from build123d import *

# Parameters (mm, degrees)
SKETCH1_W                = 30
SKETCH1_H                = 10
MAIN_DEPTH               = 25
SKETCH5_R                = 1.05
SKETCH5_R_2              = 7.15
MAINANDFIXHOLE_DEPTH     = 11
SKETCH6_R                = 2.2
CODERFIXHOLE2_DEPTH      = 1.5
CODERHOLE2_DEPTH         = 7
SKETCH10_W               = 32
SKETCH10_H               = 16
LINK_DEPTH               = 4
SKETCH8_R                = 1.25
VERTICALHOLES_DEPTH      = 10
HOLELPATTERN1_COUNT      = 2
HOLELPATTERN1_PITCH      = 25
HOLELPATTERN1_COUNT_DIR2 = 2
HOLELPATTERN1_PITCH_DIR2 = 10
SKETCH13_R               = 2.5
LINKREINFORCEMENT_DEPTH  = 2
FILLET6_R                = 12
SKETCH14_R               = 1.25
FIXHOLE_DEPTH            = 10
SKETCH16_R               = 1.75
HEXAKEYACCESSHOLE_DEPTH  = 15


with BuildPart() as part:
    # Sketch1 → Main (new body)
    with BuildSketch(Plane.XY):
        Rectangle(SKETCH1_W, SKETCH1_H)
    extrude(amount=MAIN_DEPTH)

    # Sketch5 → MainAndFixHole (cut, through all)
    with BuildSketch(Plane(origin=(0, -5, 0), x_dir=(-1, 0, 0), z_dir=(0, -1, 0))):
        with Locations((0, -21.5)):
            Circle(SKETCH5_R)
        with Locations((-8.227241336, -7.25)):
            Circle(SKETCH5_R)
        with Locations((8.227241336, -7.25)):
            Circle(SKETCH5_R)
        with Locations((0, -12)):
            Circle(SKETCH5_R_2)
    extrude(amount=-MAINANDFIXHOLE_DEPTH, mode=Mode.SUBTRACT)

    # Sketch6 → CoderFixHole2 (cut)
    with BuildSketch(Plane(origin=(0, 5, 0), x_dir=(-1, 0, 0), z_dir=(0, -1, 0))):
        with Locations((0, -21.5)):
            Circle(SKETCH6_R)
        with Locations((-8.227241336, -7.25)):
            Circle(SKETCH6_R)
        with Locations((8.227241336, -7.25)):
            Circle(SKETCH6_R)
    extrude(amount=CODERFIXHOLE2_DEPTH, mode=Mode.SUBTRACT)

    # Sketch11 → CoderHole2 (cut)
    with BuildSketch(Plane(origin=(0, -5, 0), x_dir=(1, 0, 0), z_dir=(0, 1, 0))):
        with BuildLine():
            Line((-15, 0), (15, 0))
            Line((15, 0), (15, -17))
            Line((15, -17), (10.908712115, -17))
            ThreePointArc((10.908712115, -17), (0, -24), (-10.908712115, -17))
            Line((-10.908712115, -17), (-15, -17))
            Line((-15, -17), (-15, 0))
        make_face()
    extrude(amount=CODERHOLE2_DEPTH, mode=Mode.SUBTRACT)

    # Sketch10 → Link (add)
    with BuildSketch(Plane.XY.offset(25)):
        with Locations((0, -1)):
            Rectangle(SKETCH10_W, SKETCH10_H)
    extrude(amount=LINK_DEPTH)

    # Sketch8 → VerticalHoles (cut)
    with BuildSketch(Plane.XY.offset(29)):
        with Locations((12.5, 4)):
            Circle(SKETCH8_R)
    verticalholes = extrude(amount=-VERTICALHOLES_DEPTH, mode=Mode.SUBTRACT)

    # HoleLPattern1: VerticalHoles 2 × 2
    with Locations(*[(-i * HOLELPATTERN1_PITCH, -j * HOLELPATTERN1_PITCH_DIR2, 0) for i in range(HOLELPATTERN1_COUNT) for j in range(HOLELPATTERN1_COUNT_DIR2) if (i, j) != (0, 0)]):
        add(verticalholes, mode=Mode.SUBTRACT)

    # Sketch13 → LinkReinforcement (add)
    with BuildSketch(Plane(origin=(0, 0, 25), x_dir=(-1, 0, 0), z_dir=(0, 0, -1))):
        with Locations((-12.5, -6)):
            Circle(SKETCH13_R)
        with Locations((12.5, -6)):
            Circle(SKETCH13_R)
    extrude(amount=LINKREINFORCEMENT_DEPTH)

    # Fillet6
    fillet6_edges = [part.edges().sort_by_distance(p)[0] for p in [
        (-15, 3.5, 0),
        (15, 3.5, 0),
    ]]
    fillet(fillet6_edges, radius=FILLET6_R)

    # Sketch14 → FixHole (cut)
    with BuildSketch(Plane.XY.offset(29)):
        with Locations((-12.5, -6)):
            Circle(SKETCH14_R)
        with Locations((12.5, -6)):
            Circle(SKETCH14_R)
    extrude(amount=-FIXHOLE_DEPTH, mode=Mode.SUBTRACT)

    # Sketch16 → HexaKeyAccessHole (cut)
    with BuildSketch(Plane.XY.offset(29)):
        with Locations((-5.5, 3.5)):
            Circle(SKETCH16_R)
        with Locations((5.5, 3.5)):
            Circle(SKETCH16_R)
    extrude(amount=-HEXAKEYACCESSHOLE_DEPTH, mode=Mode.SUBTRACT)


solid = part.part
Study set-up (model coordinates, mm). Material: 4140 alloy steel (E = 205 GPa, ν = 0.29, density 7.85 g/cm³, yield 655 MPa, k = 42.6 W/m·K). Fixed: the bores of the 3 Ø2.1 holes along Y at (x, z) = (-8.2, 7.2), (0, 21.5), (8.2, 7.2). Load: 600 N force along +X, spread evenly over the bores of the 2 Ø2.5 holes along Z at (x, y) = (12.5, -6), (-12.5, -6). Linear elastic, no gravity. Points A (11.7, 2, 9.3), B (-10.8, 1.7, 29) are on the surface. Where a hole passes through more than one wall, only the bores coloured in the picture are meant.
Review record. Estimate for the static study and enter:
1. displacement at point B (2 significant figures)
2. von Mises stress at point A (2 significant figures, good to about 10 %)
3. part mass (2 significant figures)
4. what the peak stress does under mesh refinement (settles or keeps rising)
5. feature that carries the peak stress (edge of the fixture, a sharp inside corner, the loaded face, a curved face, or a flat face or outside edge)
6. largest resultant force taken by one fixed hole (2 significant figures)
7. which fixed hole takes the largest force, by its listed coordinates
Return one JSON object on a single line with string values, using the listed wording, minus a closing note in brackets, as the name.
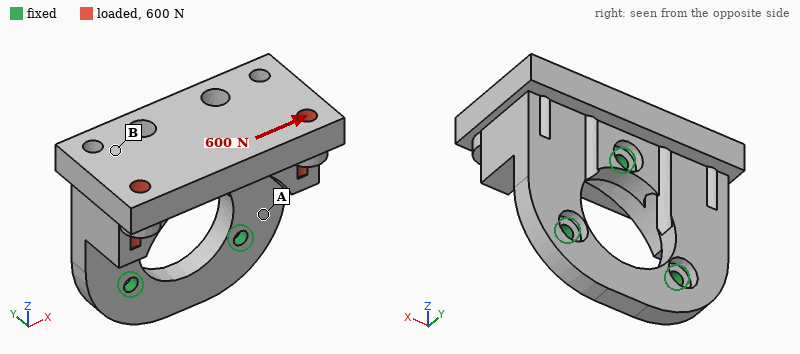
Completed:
{"displacement at point B": "23 µm", "von Mises stress at point A": "50 MPa", "part mass": "32 g", "what the peak stress does under mesh refinement": "keeps rising", "feature that carries the peak stress": "edge of the fixture", "largest resultant force taken by one fixed hole": "490 N", "which fixed hole takes the largest force, by its listed coordinates": "(0, 21.5)"}
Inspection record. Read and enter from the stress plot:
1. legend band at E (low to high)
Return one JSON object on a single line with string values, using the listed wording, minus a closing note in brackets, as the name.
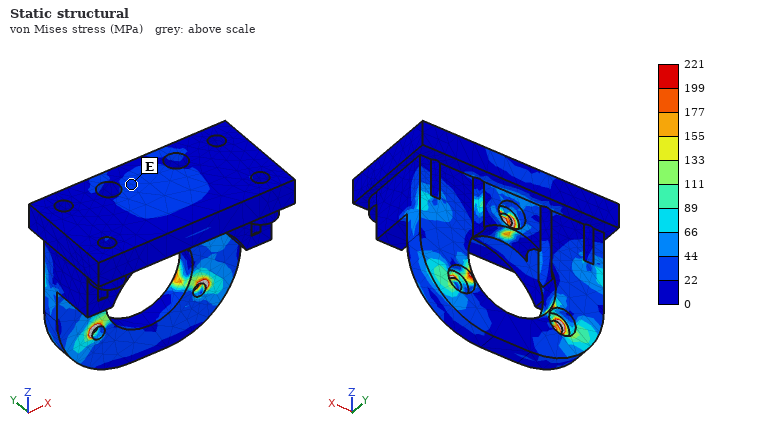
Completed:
{"legend band at E": "22 to 44 MPa"}
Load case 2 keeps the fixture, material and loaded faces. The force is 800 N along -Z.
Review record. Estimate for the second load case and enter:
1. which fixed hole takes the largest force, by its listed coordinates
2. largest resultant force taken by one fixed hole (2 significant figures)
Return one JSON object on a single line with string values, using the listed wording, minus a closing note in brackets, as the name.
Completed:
{"which fixed hole takes the largest force, by its listed coordinates": "(0, 21.5)", "largest resultant force taken by one fixed hole": "580 N"}
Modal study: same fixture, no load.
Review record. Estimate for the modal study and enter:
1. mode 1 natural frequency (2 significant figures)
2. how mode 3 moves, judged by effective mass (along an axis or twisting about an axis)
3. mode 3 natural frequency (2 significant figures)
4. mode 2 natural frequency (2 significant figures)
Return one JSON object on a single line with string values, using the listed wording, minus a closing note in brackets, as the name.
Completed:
{"mode 1 natural frequency": "4500 Hz", "how mode 3 moves, judged by effective mass": "along Y", "mode 3 natural frequency": "14 kHz", "mode 2 natural frequency": "7000 Hz"}
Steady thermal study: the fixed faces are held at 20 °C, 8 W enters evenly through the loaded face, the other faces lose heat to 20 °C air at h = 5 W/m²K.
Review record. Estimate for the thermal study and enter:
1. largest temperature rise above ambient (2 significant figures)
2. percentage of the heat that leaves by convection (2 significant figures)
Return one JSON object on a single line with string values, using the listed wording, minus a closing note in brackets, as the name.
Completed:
{"largest temperature rise above ambient": "41 K", "percentage of the heat that leaves by convection": "4.3 %"}
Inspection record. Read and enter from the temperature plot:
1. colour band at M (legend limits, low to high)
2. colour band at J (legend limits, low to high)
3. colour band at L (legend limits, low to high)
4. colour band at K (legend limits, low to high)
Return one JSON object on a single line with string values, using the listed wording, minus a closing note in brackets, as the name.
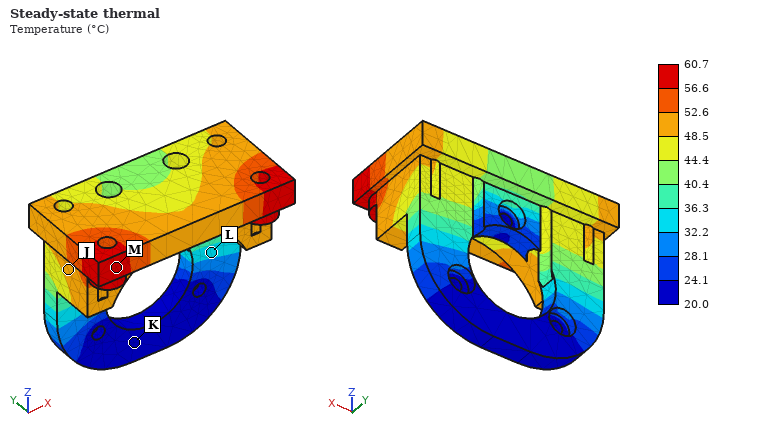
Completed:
{"colour band at M": "56.6 to 60.7 °C", "colour band at J": "48.5 to 52.6 °C", "colour band at L": "32.2 to 36.3 °C", "colour band at K": "20.0 to 24.1 °C"}
